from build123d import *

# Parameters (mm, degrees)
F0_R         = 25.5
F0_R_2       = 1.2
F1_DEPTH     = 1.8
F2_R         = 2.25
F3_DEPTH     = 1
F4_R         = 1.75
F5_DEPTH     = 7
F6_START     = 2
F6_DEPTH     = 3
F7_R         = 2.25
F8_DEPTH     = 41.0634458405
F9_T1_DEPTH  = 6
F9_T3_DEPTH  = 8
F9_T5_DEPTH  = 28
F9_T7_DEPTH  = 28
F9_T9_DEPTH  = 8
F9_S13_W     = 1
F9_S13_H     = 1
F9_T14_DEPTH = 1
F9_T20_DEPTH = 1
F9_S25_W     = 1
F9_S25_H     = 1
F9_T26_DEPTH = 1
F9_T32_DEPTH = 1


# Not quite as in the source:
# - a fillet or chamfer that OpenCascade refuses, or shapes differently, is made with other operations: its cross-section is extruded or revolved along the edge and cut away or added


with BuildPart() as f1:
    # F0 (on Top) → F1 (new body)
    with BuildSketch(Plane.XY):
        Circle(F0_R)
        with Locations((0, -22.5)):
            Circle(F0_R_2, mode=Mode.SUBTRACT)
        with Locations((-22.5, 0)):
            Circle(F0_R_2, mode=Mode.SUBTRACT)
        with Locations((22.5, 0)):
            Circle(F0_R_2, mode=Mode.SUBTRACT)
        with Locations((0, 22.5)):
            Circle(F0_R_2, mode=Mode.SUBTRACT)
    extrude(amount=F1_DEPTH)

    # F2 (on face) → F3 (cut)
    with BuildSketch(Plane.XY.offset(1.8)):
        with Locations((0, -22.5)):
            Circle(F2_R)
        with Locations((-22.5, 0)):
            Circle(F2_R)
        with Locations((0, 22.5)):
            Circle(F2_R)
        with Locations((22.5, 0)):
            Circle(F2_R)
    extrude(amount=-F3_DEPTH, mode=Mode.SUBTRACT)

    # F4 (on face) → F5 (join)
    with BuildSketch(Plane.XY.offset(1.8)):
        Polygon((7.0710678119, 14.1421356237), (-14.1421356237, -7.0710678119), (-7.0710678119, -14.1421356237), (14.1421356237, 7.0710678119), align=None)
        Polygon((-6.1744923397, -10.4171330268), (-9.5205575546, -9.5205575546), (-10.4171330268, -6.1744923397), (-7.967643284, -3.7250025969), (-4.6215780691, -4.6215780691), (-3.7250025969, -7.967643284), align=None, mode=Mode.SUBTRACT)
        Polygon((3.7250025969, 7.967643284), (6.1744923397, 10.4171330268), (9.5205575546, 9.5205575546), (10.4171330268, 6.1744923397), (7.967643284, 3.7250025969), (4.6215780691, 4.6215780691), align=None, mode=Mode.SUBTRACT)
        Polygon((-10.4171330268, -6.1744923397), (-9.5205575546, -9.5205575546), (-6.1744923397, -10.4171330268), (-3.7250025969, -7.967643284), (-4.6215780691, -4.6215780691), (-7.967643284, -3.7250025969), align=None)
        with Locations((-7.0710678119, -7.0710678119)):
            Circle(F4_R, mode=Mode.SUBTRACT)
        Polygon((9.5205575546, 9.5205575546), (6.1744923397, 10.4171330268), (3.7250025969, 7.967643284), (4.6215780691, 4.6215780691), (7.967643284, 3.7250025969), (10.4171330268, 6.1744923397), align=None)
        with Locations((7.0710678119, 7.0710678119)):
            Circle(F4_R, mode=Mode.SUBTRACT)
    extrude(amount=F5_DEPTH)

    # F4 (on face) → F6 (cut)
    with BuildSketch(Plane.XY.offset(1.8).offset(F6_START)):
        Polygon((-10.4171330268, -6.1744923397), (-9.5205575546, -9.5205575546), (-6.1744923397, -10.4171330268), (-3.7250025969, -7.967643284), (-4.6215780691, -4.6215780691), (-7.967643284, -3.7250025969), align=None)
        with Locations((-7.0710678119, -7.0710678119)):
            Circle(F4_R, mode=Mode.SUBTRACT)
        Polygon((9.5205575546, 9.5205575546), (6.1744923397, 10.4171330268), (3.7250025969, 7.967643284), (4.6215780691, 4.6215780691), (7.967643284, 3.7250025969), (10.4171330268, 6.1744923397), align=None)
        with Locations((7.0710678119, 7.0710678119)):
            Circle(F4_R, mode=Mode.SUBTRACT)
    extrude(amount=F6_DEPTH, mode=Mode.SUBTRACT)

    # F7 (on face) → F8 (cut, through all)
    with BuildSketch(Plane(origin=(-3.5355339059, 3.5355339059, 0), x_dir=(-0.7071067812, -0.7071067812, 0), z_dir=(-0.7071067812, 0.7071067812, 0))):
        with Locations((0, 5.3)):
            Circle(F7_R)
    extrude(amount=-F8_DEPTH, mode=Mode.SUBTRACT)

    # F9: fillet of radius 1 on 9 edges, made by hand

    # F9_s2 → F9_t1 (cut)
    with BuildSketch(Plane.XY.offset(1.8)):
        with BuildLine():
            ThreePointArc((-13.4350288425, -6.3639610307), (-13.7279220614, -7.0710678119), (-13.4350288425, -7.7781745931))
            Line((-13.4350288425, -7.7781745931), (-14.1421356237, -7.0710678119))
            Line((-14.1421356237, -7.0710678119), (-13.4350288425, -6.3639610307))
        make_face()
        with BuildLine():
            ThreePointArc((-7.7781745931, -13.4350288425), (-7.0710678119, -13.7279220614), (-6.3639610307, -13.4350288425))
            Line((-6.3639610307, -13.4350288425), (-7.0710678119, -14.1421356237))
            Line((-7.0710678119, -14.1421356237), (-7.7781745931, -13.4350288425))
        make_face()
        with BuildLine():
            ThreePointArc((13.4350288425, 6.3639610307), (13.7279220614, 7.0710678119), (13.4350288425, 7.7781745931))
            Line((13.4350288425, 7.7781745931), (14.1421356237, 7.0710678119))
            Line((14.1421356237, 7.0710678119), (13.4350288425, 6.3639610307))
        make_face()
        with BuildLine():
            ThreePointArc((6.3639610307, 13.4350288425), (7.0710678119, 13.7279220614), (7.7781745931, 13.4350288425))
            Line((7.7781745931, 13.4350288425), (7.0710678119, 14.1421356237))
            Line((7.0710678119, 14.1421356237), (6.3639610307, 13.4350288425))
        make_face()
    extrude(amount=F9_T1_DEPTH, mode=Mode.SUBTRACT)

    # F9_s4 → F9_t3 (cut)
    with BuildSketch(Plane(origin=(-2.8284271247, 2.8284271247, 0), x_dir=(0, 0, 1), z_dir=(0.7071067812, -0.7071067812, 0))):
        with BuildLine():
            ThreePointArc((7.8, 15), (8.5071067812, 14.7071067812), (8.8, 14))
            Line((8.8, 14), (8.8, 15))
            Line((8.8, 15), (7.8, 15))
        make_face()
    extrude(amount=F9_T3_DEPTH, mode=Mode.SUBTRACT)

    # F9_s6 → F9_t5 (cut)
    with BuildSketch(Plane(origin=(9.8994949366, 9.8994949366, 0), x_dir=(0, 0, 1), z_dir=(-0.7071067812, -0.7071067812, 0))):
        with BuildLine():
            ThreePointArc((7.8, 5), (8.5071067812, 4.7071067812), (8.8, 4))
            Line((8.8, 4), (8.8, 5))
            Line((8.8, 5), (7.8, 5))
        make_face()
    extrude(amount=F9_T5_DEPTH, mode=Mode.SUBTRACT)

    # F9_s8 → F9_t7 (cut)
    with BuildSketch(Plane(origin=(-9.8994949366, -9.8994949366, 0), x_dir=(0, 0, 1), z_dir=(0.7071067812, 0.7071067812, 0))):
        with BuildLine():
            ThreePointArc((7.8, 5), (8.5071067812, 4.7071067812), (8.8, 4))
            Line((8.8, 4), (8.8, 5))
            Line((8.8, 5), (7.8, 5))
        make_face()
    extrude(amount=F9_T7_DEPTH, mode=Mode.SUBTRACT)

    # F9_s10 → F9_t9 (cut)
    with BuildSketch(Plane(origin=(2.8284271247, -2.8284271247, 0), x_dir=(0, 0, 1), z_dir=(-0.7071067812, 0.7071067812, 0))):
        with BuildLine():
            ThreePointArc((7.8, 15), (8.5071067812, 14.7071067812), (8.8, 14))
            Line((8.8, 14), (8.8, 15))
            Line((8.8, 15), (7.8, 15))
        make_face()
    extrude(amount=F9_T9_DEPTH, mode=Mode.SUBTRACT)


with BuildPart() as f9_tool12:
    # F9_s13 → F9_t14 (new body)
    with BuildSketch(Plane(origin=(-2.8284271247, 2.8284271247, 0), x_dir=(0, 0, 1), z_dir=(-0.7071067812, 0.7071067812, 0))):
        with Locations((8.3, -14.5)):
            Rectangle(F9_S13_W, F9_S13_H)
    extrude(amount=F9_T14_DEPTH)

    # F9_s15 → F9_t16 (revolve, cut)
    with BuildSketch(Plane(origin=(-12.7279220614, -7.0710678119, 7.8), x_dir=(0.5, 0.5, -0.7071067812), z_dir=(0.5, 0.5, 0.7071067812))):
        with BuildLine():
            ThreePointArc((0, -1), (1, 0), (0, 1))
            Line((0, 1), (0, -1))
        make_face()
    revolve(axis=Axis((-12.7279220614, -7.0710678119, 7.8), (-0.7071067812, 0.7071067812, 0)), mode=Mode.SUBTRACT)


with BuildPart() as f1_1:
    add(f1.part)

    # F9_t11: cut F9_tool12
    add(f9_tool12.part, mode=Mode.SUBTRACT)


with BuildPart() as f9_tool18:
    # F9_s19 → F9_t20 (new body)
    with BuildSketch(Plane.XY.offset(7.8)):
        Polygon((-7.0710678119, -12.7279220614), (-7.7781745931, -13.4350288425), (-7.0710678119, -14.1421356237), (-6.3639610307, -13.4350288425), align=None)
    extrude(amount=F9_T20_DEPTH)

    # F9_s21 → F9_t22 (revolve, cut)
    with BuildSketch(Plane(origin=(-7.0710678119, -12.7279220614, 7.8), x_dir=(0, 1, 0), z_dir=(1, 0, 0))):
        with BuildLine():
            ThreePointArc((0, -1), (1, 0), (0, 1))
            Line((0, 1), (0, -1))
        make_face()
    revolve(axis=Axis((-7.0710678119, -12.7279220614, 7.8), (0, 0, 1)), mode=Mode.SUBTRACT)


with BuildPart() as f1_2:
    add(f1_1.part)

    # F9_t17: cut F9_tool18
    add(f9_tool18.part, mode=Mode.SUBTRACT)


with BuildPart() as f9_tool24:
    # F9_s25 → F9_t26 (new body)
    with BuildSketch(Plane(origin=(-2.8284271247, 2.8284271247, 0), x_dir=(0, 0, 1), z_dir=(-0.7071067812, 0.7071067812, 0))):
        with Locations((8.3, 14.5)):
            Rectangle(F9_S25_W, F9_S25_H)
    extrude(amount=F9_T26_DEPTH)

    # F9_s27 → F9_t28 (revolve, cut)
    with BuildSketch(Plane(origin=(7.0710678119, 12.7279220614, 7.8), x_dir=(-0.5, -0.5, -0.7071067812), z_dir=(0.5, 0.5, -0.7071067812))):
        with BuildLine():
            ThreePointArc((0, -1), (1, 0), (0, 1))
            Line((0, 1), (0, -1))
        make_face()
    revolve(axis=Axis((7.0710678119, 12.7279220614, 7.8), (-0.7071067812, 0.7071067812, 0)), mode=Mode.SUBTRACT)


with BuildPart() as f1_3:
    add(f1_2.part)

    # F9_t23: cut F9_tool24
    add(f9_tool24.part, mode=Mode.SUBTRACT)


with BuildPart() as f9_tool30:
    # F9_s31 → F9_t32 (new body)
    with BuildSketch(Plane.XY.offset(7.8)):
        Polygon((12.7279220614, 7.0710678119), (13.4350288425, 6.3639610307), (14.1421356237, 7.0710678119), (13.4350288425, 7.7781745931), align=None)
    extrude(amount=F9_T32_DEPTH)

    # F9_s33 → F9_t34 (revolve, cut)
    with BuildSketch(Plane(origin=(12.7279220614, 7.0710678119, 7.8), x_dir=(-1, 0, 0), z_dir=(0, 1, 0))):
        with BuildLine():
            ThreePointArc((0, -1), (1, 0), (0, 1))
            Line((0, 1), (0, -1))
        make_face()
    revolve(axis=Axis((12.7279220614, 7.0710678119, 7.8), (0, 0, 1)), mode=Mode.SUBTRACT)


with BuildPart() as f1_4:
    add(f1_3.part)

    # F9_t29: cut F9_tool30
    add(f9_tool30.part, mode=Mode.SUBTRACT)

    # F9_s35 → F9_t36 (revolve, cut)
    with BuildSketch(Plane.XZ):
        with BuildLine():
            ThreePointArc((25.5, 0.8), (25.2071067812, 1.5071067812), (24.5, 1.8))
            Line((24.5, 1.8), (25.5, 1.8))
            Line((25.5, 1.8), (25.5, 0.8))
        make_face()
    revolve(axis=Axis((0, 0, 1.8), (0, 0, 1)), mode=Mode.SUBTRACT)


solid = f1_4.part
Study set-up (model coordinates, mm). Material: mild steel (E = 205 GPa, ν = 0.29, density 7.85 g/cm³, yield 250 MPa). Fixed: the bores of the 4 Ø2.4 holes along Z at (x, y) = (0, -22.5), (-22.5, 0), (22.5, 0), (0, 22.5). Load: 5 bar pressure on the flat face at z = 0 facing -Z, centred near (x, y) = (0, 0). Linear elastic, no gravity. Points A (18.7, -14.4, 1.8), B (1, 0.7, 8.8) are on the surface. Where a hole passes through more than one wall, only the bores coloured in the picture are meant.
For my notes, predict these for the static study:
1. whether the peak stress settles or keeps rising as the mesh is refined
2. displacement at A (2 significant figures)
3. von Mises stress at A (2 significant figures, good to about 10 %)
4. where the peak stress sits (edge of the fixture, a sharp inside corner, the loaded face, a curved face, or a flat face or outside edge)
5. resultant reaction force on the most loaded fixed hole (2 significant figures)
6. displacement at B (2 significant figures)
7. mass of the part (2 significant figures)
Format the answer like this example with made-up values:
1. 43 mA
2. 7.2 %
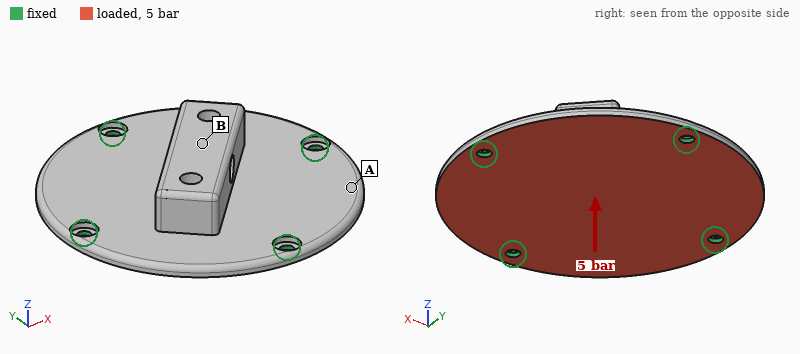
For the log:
1. keeps rising
2. 21 µm
3. 48 MPa
4. edge of the fixture
5. 400 N
6. 23 µm
7. 41 g
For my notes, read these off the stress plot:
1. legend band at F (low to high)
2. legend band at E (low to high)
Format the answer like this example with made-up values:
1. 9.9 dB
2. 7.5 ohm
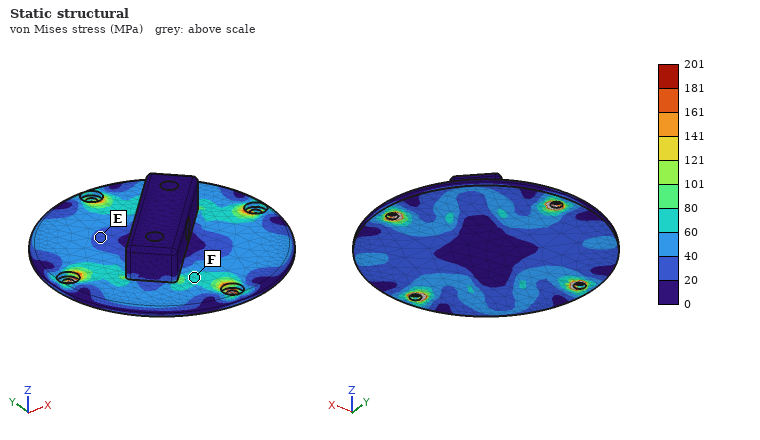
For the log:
1. 60 to 80 MPa
2. 20 to 40 MPa
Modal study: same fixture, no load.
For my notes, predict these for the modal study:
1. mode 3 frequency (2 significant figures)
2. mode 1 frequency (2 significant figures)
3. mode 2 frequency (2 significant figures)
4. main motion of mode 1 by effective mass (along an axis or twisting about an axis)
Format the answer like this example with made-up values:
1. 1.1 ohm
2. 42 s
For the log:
1. 7100 Hz
2. 4800 Hz
3. 6300 Hz
4. along Z
